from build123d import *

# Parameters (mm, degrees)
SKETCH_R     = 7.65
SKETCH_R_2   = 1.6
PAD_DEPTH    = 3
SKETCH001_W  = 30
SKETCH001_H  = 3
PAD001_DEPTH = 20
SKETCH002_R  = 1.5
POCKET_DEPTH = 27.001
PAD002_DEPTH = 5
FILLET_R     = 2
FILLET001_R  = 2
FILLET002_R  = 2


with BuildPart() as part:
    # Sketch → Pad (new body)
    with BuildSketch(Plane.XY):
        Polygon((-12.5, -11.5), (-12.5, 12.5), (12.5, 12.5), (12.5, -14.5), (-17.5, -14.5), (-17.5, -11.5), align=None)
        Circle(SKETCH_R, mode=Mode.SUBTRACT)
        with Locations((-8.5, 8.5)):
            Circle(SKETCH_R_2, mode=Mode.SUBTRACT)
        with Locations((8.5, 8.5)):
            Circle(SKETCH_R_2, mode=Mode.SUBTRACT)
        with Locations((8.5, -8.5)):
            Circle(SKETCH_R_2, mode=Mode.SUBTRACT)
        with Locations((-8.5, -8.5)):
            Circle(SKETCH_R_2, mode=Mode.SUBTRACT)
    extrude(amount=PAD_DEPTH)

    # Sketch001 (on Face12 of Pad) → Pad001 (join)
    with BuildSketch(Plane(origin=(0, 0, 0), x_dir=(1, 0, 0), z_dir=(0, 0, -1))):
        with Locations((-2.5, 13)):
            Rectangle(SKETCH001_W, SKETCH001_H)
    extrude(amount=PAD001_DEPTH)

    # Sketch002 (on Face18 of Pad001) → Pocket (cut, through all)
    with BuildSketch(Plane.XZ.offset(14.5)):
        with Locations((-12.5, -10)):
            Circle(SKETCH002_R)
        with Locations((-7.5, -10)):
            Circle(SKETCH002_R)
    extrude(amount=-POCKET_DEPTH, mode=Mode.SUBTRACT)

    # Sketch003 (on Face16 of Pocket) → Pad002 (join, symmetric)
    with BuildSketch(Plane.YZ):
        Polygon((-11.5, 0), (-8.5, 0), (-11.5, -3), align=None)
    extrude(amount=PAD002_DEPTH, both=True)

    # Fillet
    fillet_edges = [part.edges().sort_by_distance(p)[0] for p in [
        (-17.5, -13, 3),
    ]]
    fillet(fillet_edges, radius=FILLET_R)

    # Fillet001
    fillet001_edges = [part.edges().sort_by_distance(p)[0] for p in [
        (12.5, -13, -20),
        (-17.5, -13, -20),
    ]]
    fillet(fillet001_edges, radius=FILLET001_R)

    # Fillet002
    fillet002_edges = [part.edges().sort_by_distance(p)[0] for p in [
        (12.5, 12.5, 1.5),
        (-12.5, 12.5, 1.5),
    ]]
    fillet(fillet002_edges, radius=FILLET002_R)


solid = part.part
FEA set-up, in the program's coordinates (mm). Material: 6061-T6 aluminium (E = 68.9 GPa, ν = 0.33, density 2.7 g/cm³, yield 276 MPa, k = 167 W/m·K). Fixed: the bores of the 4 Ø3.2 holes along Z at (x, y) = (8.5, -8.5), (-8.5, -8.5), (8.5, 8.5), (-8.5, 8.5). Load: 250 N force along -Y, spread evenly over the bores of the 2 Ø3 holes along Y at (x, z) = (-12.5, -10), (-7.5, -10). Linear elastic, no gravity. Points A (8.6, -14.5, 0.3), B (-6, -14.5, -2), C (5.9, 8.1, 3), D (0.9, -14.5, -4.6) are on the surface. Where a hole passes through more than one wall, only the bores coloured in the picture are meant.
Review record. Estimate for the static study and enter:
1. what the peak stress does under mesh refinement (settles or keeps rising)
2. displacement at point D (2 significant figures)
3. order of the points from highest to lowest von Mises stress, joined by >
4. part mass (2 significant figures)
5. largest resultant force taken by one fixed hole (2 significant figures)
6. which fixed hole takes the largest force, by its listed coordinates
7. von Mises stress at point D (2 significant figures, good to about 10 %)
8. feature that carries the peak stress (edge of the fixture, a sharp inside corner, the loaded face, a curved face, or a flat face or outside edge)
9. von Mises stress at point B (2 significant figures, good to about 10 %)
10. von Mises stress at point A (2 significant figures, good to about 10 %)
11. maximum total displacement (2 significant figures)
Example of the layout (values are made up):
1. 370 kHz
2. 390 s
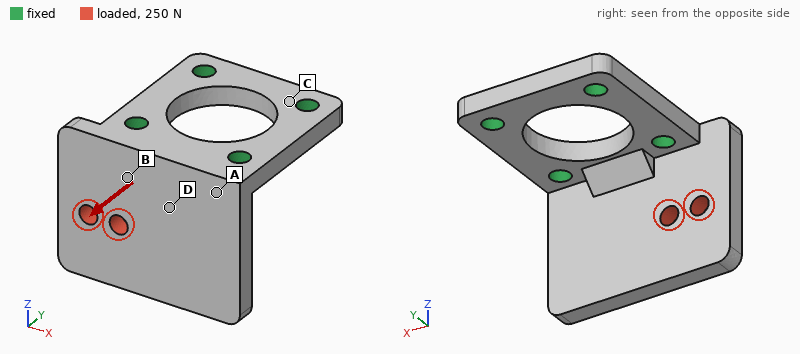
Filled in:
1. keeps rising
2. 0.021 mm
3. B > D > A > C
4. 8.7 g
5. 250 N
6. (-8.5, -8.5)
7. 39 MPa
8. edge of the fixture
9. 55 MPa
10. 25 MPa
11. 0.14 mm
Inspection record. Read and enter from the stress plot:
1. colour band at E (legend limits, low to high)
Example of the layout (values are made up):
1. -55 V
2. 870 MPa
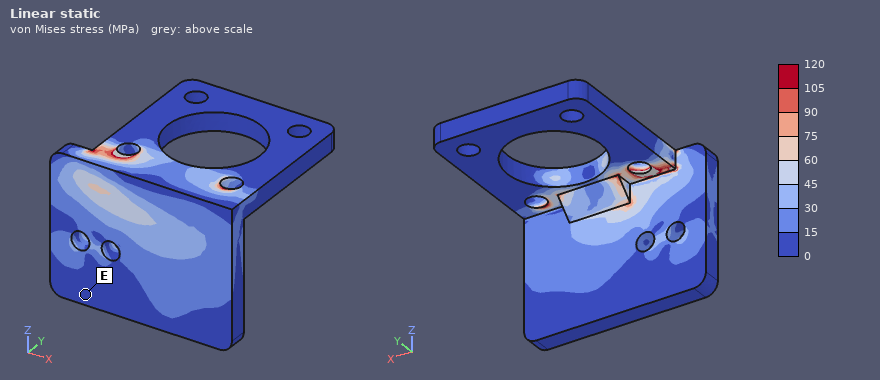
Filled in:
1. 0 to 15 MPa
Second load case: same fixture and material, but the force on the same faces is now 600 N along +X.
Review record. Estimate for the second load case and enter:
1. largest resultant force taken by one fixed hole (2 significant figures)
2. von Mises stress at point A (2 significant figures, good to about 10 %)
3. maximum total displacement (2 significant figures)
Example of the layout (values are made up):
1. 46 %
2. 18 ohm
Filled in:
1. 510 N
2. 10 MPa
3. 24 µm
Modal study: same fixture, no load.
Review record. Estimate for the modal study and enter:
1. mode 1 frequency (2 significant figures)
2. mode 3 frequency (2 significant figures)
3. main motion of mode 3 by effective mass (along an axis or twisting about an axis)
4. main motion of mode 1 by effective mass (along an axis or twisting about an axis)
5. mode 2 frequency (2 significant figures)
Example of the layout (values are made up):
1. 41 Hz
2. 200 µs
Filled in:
1. 4400 Hz
2. 15 kHz
3. along X
4. along Y
5. 8500 Hz
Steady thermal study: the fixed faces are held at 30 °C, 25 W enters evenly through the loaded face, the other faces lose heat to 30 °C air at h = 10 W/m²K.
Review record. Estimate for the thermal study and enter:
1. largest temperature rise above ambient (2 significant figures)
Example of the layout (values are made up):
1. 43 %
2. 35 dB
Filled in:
1. 41 K
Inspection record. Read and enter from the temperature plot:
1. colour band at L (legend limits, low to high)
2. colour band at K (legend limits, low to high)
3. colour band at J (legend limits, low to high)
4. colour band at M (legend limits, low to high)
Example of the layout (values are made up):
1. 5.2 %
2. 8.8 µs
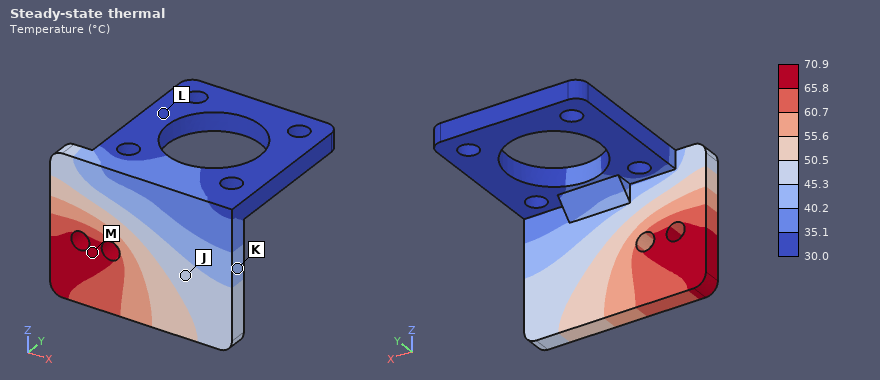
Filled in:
1. 30.0 to 35.1 °C
2. 40.2 to 45.3 °C
3. 45.3 to 50.5 °C
4. 65.8 to 70.9 °C
